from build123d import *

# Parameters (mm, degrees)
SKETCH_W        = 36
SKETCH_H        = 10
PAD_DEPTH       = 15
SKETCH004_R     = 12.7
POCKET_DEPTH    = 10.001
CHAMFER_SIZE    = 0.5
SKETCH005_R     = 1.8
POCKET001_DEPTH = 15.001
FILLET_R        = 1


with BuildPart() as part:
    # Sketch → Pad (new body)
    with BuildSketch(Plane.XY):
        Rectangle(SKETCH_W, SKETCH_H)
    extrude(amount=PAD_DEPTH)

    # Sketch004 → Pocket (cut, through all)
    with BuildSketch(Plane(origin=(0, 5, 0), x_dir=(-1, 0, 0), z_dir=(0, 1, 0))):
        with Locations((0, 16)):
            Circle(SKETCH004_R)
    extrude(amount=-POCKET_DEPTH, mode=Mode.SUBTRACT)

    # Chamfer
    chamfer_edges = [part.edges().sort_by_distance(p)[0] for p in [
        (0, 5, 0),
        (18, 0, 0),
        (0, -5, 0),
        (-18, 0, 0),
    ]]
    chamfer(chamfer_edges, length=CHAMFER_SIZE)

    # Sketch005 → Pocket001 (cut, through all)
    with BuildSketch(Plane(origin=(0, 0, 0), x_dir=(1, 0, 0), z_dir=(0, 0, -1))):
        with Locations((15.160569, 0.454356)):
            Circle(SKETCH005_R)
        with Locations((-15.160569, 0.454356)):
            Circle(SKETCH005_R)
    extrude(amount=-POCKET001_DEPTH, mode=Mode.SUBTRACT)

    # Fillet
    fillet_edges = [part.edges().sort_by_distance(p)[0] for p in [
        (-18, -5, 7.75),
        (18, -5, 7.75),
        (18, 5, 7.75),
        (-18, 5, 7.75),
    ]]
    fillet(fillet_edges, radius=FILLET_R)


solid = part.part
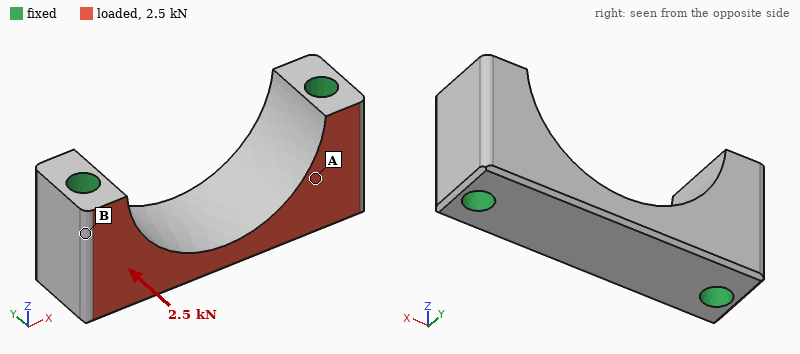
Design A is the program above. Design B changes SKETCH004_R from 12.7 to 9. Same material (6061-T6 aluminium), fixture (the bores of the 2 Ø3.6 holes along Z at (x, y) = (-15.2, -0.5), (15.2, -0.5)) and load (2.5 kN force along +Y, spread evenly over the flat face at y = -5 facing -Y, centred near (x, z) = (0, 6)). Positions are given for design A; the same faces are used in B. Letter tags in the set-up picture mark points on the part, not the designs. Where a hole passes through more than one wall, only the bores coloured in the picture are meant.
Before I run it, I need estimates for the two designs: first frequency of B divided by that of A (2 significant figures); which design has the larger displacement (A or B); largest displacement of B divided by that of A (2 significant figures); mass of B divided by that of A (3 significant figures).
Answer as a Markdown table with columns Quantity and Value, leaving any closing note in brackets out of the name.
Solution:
| Quantity | Value |
|---|---|
| first frequency of B divided by that of A | 0.91 |
| which design has the larger displacement | A |
| largest displacement of B divided by that of A | 0.86 |
| mass of B divided by that of A | 1.43 |
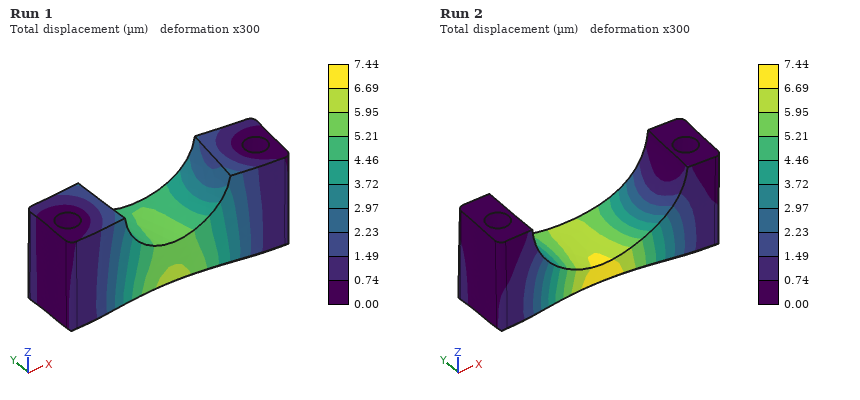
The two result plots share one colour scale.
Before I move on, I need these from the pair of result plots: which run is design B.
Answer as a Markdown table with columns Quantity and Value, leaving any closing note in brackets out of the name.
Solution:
| Quantity | Value |
|---|---|
| which run is design B | Run 1 |
